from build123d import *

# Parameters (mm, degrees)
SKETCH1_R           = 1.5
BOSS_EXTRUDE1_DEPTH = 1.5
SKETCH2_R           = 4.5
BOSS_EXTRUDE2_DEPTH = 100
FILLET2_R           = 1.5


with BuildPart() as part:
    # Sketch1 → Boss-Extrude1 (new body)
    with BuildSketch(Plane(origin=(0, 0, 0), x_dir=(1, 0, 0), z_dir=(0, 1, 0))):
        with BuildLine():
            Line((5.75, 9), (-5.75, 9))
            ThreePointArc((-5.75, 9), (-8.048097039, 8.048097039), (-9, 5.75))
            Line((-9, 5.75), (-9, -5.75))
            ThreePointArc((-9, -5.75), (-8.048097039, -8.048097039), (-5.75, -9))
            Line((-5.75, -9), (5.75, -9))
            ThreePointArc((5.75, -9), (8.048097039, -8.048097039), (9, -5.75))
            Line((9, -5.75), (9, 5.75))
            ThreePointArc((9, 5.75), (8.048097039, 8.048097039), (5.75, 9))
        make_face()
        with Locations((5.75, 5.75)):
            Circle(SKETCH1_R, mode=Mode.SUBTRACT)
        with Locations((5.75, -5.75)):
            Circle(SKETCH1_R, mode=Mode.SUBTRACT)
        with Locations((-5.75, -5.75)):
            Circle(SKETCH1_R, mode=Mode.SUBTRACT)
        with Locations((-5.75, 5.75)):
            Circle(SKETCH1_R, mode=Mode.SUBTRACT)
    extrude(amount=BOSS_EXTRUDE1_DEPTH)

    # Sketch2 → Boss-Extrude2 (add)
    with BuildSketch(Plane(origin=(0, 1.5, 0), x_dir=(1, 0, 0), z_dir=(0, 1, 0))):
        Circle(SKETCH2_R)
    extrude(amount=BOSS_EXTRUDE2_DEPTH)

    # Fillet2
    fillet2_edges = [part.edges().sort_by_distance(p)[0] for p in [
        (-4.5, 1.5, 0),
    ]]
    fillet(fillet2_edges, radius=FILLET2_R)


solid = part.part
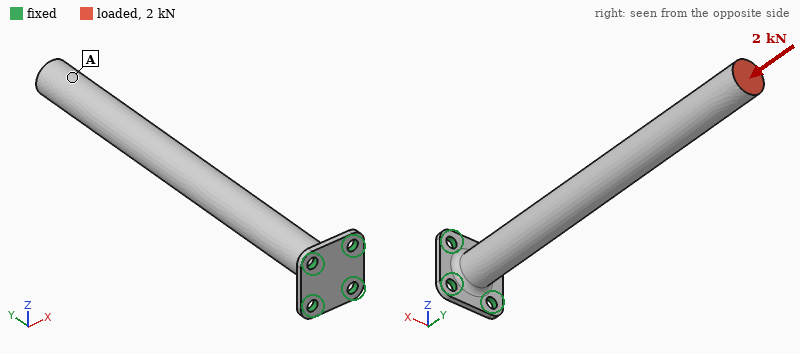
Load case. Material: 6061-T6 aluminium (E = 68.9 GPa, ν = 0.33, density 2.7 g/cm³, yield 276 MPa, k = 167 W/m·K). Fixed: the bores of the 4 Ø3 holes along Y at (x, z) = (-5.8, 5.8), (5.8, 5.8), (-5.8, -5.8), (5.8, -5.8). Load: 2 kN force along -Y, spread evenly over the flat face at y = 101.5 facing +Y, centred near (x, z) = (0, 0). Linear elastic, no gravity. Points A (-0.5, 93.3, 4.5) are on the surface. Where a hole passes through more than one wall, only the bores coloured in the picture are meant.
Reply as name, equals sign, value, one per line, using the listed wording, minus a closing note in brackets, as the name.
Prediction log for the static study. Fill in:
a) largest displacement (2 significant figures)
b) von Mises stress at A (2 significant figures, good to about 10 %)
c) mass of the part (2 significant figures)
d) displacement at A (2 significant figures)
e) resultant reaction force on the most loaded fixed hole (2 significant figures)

largest displacement = 60 µm
von Mises stress at A = 31 MPa
mass of the part = 18 g
displacement at A = 56 µm
resultant reaction force on the most loaded fixed hole = 560 N
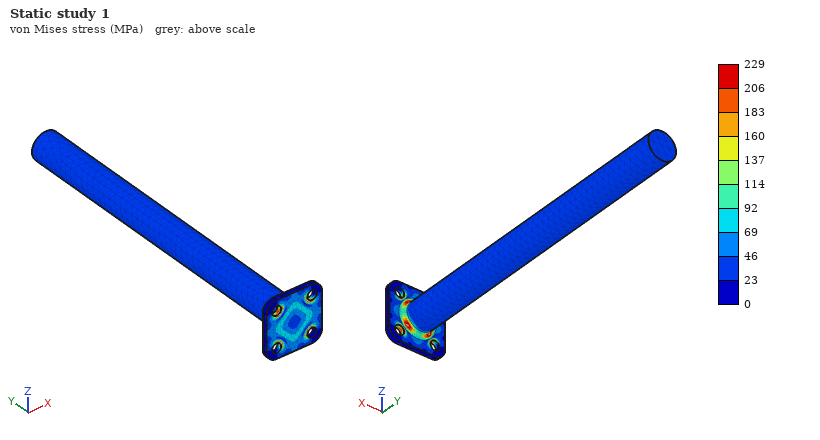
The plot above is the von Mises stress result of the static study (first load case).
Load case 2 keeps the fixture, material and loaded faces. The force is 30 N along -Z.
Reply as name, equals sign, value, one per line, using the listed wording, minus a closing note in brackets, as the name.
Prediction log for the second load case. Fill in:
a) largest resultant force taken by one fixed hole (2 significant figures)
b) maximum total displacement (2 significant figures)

largest resultant force taken by one fixed hole = 160 N
maximum total displacement = 0.56 mm
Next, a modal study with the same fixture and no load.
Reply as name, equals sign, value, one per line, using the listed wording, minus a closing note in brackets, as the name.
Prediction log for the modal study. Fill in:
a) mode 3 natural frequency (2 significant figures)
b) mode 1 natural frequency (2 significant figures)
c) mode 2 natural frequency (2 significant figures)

mode 3 natural frequency = 3500 Hz
mode 1 natural frequency = 550 Hz
mode 2 natural frequency = 550 Hz
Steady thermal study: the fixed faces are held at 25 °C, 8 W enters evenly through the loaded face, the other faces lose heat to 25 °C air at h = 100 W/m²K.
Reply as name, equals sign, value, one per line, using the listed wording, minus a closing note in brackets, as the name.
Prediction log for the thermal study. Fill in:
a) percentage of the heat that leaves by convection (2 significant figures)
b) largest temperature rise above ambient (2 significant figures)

percentage of the heat that leaves by convection = 65 %
largest temperature rise above ambient = 43 K
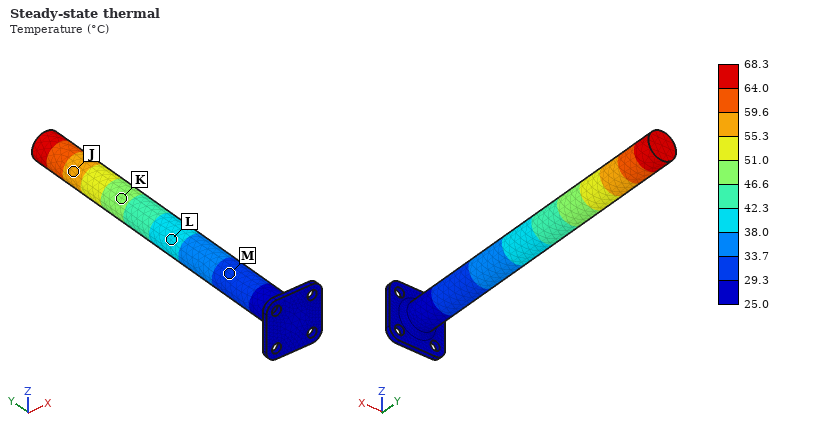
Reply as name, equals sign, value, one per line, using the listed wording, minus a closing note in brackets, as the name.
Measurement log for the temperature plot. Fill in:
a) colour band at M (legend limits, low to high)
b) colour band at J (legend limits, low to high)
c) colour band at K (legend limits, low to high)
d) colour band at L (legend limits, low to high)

colour band at M = 29.3 to 33.7 °C
colour band at J = 55.3 to 59.6 °C
colour band at K = 46.6 to 51.0 °C
colour band at L = 38.0 to 42.3 °C
